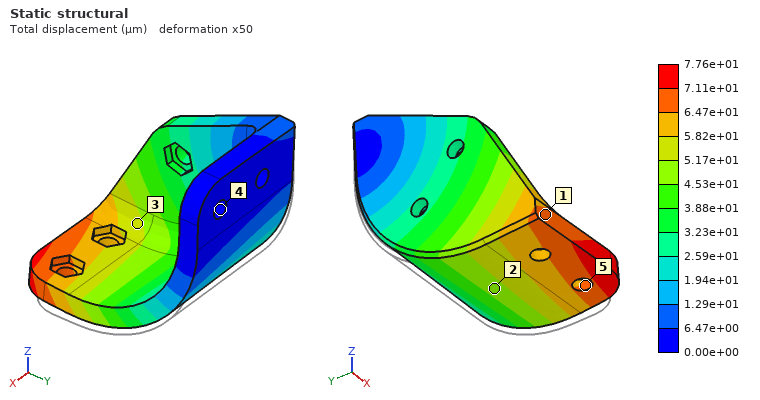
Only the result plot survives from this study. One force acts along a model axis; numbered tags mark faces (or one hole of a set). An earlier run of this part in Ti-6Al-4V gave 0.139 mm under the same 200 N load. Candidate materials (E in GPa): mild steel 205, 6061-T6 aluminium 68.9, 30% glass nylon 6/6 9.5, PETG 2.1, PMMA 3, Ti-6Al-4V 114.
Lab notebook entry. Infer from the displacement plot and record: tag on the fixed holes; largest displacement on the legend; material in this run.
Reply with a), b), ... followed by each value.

a) 4
b) 7.76e+01 µm
c) mild steel
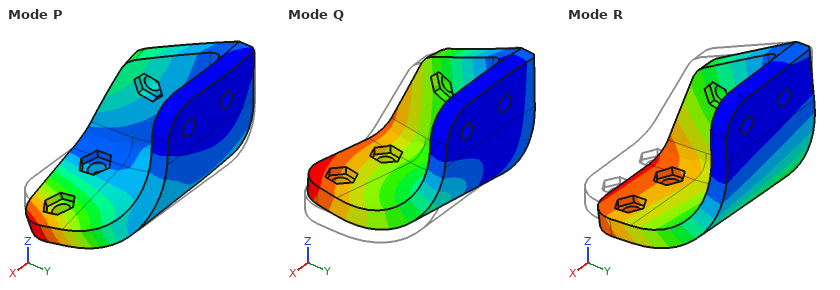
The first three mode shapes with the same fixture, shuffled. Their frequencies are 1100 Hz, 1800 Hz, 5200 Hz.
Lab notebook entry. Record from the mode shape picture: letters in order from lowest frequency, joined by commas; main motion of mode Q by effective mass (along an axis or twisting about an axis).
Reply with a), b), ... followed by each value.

a) R, Q, P
b) along X
